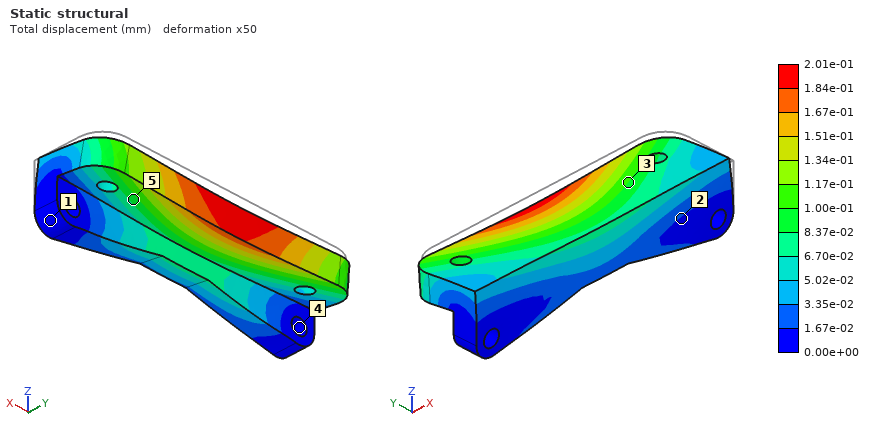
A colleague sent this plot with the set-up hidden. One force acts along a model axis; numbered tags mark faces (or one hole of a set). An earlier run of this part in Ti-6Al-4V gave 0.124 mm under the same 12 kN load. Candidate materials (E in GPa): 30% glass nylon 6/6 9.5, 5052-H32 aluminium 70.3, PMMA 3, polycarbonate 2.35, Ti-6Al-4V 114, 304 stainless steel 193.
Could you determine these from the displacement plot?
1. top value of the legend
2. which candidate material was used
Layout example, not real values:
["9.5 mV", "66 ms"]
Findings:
["2.01e-01 mm", "5052-H32 aluminium"]
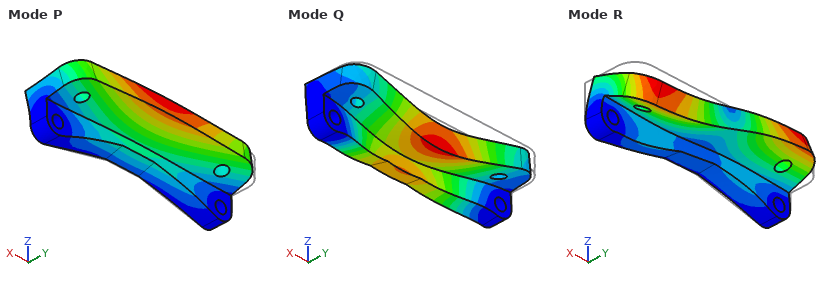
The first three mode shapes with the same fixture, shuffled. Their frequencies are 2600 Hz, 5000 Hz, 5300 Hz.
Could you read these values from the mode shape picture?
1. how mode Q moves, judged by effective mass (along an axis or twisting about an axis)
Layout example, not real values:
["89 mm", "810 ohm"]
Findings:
["along Y"]
